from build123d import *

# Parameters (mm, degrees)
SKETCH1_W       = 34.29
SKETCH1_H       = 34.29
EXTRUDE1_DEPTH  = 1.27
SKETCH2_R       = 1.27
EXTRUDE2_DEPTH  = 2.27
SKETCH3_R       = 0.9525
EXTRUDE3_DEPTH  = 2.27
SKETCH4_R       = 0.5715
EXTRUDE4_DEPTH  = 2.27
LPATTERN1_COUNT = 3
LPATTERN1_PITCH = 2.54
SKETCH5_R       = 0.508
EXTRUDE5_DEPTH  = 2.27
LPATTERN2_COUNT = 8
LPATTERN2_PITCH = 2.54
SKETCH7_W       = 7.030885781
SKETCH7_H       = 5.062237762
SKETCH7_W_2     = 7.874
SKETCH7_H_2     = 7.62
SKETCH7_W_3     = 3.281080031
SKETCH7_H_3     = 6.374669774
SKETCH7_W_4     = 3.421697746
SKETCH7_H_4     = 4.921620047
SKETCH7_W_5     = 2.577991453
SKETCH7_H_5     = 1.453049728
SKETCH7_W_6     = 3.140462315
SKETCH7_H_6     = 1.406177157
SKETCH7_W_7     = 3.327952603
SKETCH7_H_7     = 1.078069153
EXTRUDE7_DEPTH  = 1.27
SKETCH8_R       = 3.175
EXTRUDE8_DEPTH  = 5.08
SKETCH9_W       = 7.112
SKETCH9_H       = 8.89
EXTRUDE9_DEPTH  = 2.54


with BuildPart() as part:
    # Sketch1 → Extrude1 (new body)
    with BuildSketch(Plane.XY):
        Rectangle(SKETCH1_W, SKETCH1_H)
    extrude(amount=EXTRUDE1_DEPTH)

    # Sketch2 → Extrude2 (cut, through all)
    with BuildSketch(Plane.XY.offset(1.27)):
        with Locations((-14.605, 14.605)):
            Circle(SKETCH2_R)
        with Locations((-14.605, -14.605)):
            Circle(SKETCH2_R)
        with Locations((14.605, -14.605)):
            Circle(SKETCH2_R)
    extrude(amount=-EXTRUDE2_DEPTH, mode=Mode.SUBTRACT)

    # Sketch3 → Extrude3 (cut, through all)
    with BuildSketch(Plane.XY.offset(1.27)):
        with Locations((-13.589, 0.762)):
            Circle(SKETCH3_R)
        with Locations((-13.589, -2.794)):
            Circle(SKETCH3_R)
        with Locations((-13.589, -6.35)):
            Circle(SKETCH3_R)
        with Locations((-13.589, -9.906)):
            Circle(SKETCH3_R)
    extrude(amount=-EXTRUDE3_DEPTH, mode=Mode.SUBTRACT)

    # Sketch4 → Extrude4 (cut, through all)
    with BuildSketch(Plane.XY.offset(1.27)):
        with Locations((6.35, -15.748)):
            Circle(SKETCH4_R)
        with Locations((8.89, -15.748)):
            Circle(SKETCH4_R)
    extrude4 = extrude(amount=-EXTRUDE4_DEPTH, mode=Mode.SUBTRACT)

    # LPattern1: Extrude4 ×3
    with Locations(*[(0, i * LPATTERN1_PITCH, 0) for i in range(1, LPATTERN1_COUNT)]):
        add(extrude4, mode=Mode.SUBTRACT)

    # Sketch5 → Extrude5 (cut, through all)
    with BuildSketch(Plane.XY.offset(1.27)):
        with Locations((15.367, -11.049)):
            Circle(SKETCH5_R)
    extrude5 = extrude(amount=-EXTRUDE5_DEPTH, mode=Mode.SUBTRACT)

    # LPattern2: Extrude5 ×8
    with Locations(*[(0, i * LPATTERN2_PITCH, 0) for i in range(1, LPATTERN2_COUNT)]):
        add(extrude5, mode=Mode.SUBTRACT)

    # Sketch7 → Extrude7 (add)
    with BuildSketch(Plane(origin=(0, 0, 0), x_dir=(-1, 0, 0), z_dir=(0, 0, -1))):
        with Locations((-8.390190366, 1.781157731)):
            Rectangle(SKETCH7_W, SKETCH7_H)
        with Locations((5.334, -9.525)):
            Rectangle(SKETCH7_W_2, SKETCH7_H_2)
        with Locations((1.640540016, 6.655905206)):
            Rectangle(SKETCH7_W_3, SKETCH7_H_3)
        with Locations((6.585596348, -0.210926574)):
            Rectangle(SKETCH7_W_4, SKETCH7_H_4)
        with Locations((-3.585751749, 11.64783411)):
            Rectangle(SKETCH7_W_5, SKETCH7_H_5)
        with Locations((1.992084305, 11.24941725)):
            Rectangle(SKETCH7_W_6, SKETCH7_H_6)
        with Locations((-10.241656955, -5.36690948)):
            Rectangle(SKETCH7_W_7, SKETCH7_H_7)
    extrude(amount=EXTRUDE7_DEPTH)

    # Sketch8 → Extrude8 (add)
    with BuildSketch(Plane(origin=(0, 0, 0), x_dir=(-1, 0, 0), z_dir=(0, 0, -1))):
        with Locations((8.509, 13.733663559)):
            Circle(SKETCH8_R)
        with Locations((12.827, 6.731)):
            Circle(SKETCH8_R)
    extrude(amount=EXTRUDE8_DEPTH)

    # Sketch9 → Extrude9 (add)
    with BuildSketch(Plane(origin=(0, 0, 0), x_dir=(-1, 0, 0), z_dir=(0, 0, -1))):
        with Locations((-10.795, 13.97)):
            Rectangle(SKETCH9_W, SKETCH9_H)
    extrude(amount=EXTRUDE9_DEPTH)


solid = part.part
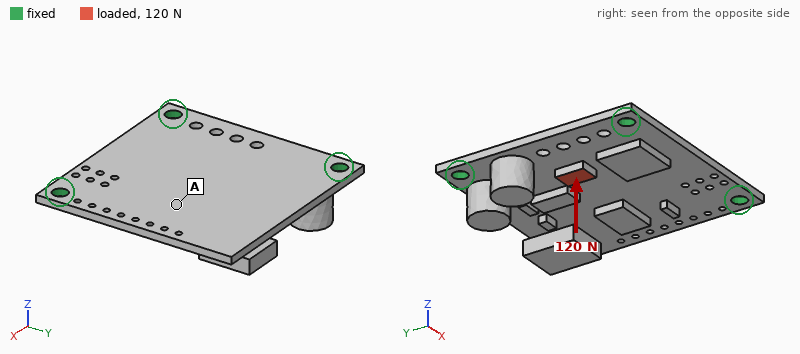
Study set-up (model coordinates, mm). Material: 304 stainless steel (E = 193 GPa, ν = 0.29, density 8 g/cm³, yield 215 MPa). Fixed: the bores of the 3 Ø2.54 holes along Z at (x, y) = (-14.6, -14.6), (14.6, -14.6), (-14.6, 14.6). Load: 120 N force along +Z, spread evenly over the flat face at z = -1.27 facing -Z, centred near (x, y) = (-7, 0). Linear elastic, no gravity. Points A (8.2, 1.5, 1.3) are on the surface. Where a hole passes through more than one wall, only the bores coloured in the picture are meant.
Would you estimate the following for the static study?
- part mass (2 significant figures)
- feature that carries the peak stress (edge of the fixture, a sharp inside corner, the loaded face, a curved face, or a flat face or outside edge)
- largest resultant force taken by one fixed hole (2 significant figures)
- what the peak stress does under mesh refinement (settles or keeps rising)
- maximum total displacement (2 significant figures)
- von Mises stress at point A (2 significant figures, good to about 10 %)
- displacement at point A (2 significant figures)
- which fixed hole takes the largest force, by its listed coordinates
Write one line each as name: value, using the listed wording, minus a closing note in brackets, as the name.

part mass: 17 g
feature that carries the peak stress: edge of the fixture
largest resultant force taken by one fixed hole: 55 N
what the peak stress does under mesh refinement: keeps rising
maximum total displacement: 31 µm
von Mises stress at point A: 15 MPa
displacement at point A: 24 µm
which fixed hole takes the largest force, by its listed coordinates: (-14.6, 14.6)
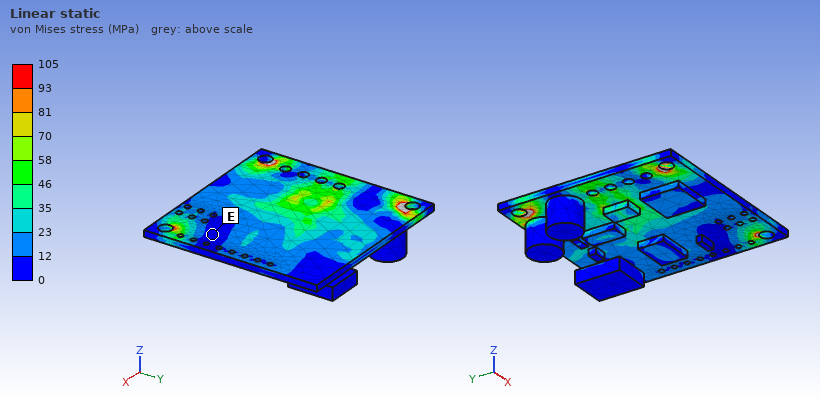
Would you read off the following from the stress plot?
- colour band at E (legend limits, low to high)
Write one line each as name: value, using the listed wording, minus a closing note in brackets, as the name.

colour band at E: 0 to 12 MPa
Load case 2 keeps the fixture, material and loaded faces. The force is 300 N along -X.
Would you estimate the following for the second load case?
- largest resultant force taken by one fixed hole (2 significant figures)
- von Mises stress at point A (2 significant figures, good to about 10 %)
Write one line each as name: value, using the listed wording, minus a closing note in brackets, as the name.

largest resultant force taken by one fixed hole: 130 N
von Mises stress at point A: 8.8 MPa
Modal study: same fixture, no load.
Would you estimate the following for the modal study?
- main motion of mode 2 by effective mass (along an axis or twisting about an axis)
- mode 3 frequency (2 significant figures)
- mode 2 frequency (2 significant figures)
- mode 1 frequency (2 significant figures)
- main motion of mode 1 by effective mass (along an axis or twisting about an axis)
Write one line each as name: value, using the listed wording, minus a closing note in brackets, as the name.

main motion of mode 2 by effective mass: along Z
mode 3 frequency: 6800 Hz
mode 2 frequency: 4900 Hz
mode 1 frequency: 1800 Hz
main motion of mode 1 by effective mass: along Z
